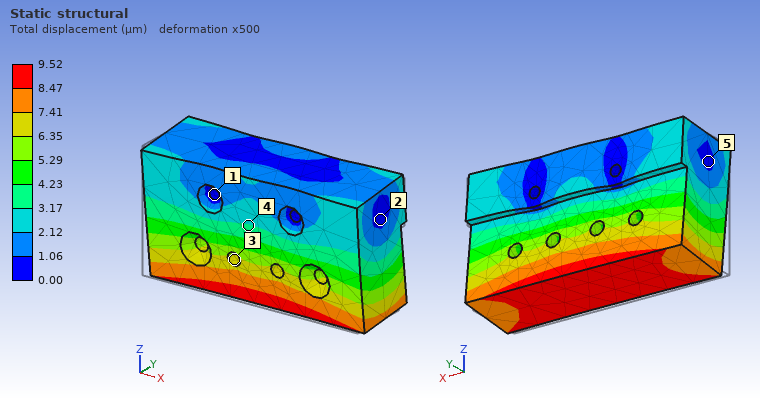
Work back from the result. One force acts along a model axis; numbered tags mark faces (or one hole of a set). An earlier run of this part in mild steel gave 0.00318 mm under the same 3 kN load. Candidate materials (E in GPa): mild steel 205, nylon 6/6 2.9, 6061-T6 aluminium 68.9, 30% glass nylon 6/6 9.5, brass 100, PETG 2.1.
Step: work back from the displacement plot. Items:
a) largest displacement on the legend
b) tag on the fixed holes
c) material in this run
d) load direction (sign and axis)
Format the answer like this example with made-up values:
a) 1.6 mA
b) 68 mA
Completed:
a) 9.52 µm
b) 1
c) 6061-T6 aluminium
d) +Y
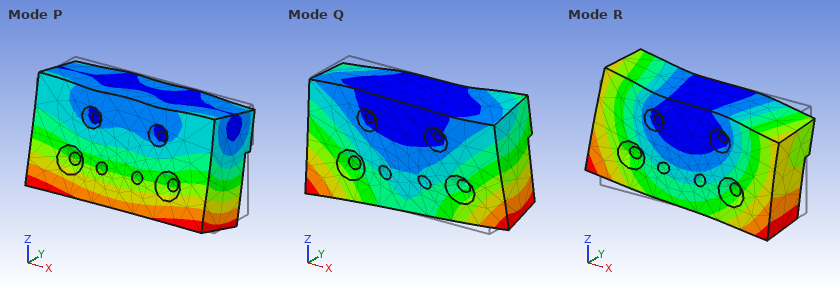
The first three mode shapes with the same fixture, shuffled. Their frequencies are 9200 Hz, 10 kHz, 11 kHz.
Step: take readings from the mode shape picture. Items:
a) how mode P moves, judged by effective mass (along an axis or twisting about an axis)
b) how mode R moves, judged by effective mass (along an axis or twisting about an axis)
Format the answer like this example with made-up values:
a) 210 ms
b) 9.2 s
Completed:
a) along Y
b) along X
